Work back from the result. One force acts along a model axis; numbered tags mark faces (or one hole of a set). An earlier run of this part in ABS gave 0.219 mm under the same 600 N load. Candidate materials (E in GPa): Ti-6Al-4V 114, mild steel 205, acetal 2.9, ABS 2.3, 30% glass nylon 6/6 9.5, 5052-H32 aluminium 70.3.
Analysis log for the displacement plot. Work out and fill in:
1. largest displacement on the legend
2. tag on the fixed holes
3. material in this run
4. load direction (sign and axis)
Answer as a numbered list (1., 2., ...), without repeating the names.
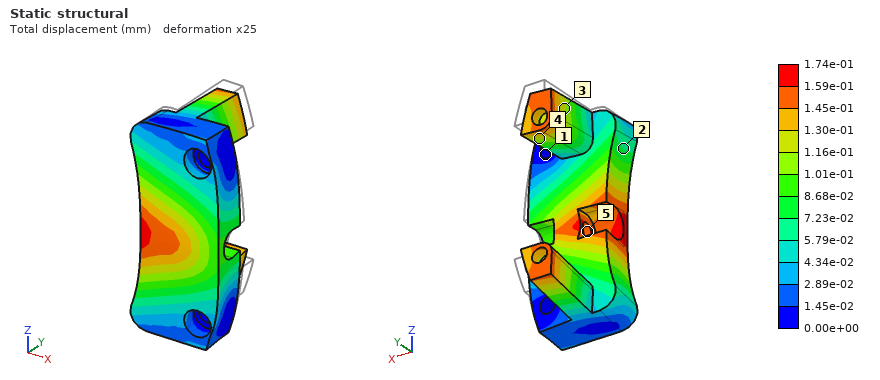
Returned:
1. 1.74e-01 mm
2. 1
3. acetal
4. -Y
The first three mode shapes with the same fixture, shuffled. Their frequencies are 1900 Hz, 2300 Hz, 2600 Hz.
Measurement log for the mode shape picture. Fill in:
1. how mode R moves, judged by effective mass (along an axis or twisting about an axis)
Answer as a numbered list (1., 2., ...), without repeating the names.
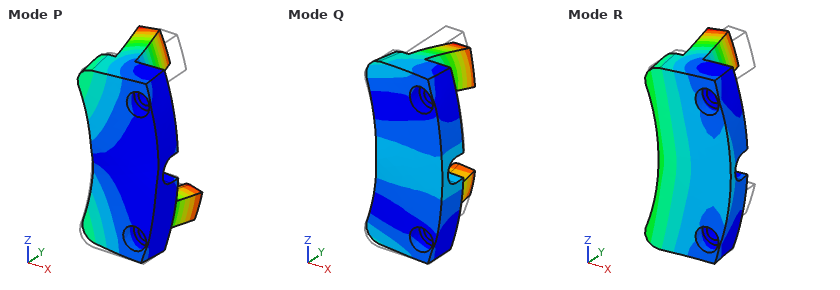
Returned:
1. along Y
